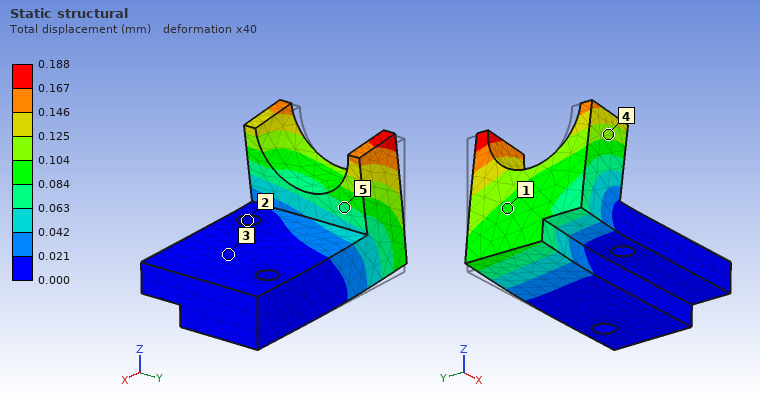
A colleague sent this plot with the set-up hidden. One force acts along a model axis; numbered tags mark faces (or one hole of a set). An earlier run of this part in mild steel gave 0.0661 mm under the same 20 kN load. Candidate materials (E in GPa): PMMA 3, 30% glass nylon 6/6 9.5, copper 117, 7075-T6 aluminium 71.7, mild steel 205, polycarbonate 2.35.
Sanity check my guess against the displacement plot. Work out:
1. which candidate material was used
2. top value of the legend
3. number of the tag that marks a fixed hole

7075-T6 aluminium
0.188 mm
2
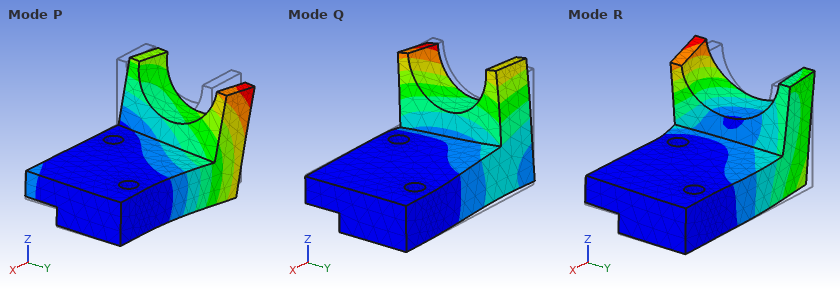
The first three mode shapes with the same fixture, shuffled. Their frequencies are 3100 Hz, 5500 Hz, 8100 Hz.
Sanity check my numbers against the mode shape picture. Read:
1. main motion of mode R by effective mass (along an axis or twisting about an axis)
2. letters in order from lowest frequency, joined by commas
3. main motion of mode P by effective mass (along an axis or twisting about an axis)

along Y
P, Q, R
along Z
